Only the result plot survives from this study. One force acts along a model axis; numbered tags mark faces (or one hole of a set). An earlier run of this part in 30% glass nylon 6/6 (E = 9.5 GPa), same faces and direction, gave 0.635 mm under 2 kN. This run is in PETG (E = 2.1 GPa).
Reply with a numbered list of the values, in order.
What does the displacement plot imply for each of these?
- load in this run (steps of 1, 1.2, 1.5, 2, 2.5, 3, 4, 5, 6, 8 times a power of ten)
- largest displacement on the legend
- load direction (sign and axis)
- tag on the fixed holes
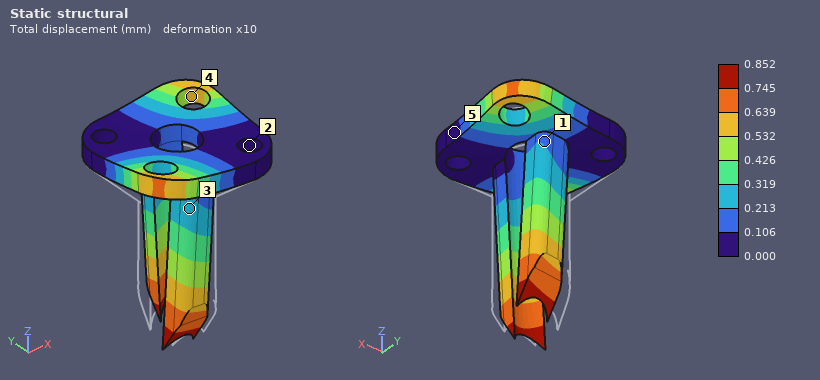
1. 600 N
2. 0.852 mm
3. +Z
4. 2
